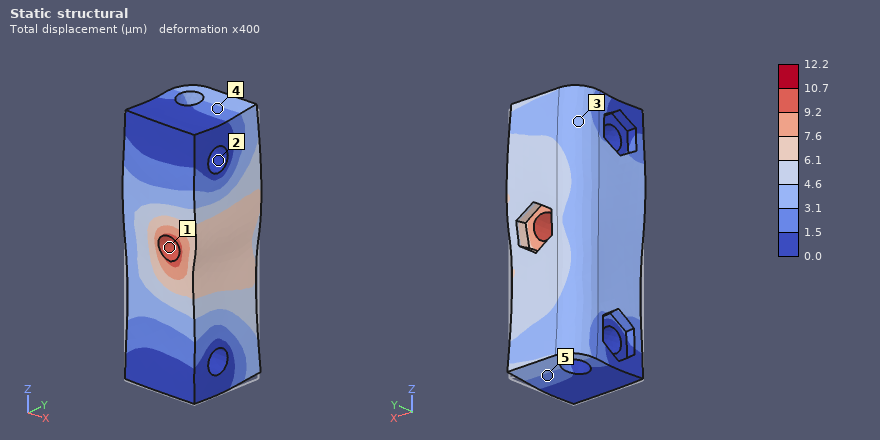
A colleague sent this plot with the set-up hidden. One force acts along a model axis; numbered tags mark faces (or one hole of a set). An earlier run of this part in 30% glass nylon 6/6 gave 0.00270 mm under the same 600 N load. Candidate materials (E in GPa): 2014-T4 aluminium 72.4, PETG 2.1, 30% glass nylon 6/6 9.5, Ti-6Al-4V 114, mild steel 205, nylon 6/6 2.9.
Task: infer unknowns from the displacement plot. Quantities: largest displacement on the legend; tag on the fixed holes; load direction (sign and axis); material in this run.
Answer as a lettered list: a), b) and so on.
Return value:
a) 12.2 µm
b) 2
c) +Z
d) PETG
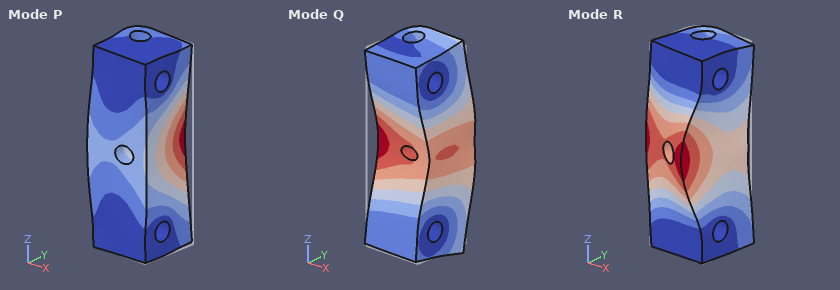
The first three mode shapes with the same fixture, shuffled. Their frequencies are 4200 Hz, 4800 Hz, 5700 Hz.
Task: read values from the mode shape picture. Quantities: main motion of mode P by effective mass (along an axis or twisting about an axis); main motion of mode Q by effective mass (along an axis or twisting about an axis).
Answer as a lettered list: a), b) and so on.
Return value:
a) along X
b) along Y
